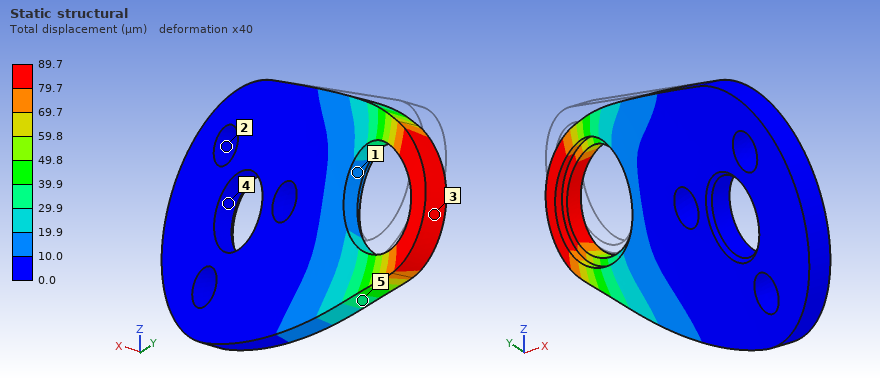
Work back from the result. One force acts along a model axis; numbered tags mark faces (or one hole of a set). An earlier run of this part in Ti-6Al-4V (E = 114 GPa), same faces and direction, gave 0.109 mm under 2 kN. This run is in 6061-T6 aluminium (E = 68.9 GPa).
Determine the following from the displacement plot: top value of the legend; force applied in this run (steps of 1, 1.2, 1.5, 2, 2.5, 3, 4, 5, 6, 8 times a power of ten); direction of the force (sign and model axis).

89.7 µm
1 kN
-Z
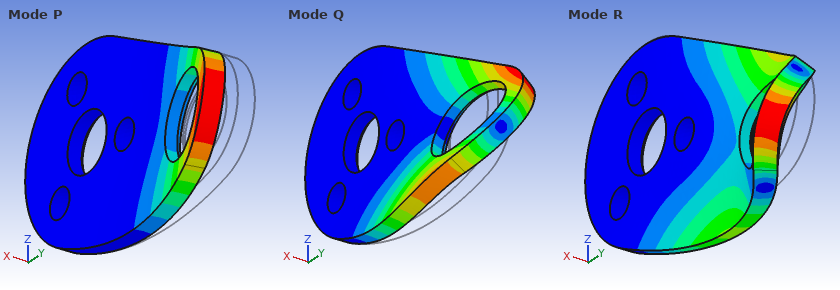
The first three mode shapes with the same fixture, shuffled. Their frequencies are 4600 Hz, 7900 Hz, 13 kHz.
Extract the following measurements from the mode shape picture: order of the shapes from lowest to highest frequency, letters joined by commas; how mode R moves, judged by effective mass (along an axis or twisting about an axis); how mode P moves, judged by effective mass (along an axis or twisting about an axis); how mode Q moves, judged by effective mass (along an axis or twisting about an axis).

P, Q, R
along X
along X
twisting about Y
